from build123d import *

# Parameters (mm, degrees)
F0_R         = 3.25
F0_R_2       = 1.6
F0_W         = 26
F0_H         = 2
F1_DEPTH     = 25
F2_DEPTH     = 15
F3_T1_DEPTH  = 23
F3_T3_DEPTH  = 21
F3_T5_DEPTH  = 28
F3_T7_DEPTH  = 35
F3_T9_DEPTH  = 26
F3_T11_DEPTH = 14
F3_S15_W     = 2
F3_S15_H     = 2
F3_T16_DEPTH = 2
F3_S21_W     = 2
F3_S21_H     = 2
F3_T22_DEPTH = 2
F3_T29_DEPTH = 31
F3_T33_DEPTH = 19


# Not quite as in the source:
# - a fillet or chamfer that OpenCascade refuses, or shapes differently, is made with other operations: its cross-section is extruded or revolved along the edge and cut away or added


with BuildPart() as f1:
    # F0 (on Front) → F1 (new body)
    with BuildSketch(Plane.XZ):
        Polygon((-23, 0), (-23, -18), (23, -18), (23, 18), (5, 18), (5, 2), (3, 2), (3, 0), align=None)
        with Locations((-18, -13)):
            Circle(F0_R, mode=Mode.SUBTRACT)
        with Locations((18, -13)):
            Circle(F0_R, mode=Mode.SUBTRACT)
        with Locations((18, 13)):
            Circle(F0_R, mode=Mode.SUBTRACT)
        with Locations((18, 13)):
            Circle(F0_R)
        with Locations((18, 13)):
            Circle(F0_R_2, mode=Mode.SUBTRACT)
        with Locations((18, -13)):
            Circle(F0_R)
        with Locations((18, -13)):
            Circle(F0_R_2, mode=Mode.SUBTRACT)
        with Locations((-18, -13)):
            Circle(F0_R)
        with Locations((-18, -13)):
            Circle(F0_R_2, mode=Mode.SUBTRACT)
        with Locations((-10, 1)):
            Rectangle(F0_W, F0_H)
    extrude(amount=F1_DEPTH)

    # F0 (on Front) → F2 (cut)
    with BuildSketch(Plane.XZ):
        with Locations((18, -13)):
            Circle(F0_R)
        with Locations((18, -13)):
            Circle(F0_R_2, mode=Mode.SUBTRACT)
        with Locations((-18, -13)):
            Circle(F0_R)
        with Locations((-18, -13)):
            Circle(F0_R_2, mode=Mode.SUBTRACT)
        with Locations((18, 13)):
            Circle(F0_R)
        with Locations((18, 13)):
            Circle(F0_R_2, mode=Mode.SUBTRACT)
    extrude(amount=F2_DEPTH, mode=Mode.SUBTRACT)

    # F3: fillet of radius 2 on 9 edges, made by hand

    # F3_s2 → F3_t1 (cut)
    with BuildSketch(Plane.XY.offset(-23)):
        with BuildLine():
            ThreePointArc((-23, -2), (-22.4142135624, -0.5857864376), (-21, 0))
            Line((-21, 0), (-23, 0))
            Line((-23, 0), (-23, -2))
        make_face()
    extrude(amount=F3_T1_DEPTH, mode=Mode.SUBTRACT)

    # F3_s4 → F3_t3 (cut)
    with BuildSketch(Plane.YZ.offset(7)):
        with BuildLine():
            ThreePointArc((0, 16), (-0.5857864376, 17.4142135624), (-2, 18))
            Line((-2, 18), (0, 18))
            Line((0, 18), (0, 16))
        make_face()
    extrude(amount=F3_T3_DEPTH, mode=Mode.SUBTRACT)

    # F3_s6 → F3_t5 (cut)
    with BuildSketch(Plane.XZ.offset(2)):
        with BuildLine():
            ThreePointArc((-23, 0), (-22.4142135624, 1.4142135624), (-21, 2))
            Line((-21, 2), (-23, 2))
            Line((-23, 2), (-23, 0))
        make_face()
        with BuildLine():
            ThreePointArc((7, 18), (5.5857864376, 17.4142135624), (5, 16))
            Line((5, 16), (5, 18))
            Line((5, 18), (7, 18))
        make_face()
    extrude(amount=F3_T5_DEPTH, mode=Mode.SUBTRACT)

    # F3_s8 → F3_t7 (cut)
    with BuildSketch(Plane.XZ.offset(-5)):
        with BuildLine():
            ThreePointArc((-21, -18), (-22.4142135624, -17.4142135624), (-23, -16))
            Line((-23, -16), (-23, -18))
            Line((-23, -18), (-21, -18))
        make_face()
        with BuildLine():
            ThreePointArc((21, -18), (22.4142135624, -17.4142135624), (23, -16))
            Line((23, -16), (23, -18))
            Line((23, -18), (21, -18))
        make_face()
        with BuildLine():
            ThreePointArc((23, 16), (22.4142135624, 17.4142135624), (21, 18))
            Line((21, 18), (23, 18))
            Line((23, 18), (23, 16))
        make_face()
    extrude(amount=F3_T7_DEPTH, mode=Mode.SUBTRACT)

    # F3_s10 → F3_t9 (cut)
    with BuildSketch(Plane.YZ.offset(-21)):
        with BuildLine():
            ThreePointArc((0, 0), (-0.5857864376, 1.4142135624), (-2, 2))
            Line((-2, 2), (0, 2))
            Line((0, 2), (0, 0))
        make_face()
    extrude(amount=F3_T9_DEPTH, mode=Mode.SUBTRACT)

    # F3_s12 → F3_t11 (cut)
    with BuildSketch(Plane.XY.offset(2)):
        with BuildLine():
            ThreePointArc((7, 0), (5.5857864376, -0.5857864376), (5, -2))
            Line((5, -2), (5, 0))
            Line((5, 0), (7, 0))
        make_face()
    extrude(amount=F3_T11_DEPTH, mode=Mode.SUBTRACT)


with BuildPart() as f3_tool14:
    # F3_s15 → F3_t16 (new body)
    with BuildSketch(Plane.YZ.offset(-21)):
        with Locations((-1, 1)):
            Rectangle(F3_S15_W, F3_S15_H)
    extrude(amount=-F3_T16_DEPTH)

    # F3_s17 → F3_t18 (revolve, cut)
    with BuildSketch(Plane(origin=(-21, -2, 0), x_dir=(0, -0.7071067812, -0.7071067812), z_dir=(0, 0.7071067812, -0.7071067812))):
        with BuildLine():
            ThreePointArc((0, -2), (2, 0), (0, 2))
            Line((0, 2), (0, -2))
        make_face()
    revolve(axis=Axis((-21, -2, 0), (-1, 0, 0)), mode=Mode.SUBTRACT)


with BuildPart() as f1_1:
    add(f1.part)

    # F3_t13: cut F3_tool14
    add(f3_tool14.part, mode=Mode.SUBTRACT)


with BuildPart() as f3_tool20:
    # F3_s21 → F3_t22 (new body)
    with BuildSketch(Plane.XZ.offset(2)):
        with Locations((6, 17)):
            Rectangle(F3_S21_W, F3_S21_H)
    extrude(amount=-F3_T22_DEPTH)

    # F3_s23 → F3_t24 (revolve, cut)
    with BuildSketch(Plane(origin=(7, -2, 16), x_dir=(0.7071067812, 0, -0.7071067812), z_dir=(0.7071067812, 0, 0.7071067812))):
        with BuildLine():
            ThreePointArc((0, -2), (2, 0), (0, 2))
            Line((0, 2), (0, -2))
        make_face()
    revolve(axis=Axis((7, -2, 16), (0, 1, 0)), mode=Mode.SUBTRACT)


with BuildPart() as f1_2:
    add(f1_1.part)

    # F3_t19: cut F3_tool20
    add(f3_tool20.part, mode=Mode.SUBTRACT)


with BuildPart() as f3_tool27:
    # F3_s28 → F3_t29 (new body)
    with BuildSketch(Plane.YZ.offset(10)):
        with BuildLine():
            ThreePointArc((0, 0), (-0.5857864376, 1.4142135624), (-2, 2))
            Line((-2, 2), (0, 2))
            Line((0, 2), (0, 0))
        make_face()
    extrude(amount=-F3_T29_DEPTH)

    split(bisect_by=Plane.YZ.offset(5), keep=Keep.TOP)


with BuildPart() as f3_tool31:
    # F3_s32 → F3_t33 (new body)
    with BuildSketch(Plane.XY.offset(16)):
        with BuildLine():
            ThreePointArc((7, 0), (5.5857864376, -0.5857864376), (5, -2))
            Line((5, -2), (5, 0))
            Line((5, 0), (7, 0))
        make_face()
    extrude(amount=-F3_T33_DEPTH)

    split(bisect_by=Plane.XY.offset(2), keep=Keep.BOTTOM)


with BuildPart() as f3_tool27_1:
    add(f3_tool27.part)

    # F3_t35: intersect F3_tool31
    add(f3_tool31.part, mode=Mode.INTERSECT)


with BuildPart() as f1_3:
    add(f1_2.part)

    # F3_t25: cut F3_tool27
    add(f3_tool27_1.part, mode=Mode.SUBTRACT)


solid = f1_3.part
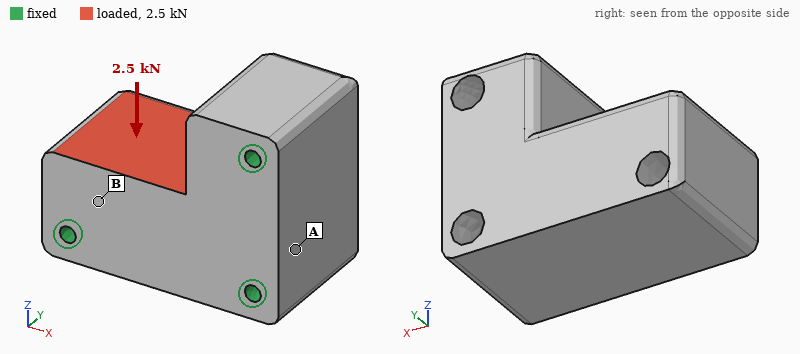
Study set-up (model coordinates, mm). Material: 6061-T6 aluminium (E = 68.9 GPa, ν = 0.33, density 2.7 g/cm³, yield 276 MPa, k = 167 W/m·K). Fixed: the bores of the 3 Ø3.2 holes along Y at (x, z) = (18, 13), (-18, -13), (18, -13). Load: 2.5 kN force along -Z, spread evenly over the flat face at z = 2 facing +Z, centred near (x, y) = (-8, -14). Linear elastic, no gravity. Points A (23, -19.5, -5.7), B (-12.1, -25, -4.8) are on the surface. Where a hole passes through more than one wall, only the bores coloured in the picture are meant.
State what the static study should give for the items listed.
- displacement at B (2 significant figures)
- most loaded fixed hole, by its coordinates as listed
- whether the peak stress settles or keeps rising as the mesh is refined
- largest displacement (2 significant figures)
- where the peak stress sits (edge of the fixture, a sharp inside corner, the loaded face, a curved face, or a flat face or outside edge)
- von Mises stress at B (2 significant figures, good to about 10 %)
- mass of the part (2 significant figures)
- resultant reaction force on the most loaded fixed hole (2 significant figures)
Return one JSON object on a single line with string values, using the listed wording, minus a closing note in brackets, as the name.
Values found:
{"displacement at B": "1.3 µm", "most loaded fixed hole, by its coordinates as listed": "(-18, -13)", "whether the peak stress settles or keeps rising as the mesh is refined": "keeps rising", "largest displacement": "6.9 µm", "where the peak stress sits": "edge of the fixture", "von Mises stress at B": "7.3 MPa", "mass of the part": "76 g", "resultant reaction force on the most loaded fixed hole": "1.4 kN"}
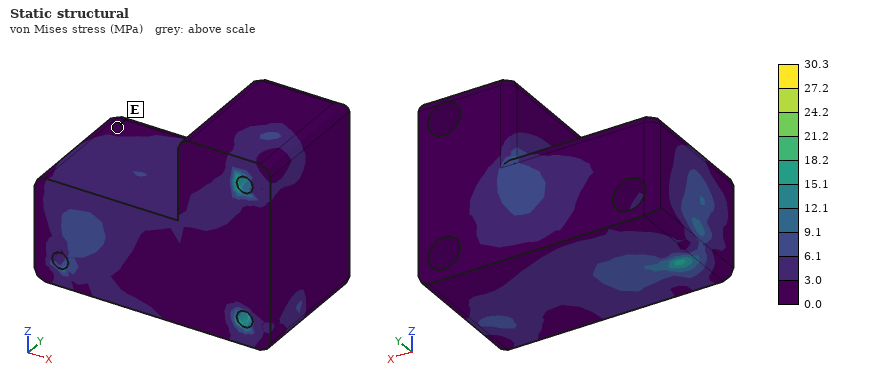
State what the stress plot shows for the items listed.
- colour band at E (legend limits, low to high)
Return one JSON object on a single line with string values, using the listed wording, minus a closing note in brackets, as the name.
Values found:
{"colour band at E": "0.0 to 3.0 MPa"}
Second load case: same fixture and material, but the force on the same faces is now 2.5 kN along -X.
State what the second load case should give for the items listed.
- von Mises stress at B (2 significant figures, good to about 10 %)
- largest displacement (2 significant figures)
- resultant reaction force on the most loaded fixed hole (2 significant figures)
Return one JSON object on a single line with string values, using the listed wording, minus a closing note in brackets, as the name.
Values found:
{"von Mises stress at B": "6.4 MPa", "largest displacement": "5.6 µm", "resultant reaction force on the most loaded fixed hole": "1.4 kN"}
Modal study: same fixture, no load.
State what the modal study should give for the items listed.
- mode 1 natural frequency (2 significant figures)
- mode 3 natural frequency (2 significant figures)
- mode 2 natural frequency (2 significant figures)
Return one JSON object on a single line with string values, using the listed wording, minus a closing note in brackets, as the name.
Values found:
{"mode 1 natural frequency": "15 kHz", "mode 3 natural frequency": "23 kHz", "mode 2 natural frequency": "22 kHz"}
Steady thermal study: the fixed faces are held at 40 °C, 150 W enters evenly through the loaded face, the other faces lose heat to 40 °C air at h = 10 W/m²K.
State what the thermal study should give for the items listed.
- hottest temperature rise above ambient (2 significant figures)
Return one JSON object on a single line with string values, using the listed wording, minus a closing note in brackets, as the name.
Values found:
{"hottest temperature rise above ambient": "32 K"}
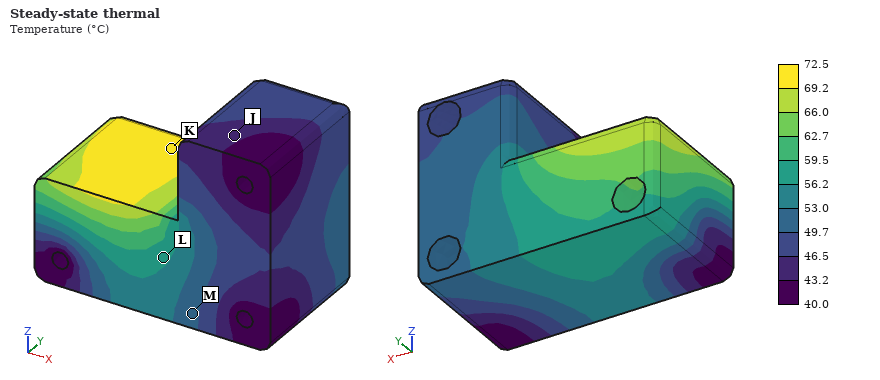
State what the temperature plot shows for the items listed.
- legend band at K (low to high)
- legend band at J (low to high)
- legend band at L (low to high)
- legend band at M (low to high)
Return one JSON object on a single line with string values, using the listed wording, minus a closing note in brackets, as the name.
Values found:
{"legend band at K": "69.2 to 72.5 °C", "legend band at J": "43.2 to 46.5 °C", "legend band at L": "56.2 to 59.5 °C", "legend band at M": "49.7 to 53.0 °C"}
